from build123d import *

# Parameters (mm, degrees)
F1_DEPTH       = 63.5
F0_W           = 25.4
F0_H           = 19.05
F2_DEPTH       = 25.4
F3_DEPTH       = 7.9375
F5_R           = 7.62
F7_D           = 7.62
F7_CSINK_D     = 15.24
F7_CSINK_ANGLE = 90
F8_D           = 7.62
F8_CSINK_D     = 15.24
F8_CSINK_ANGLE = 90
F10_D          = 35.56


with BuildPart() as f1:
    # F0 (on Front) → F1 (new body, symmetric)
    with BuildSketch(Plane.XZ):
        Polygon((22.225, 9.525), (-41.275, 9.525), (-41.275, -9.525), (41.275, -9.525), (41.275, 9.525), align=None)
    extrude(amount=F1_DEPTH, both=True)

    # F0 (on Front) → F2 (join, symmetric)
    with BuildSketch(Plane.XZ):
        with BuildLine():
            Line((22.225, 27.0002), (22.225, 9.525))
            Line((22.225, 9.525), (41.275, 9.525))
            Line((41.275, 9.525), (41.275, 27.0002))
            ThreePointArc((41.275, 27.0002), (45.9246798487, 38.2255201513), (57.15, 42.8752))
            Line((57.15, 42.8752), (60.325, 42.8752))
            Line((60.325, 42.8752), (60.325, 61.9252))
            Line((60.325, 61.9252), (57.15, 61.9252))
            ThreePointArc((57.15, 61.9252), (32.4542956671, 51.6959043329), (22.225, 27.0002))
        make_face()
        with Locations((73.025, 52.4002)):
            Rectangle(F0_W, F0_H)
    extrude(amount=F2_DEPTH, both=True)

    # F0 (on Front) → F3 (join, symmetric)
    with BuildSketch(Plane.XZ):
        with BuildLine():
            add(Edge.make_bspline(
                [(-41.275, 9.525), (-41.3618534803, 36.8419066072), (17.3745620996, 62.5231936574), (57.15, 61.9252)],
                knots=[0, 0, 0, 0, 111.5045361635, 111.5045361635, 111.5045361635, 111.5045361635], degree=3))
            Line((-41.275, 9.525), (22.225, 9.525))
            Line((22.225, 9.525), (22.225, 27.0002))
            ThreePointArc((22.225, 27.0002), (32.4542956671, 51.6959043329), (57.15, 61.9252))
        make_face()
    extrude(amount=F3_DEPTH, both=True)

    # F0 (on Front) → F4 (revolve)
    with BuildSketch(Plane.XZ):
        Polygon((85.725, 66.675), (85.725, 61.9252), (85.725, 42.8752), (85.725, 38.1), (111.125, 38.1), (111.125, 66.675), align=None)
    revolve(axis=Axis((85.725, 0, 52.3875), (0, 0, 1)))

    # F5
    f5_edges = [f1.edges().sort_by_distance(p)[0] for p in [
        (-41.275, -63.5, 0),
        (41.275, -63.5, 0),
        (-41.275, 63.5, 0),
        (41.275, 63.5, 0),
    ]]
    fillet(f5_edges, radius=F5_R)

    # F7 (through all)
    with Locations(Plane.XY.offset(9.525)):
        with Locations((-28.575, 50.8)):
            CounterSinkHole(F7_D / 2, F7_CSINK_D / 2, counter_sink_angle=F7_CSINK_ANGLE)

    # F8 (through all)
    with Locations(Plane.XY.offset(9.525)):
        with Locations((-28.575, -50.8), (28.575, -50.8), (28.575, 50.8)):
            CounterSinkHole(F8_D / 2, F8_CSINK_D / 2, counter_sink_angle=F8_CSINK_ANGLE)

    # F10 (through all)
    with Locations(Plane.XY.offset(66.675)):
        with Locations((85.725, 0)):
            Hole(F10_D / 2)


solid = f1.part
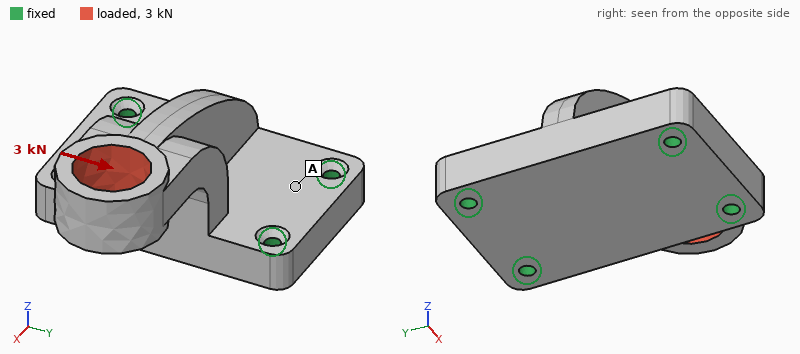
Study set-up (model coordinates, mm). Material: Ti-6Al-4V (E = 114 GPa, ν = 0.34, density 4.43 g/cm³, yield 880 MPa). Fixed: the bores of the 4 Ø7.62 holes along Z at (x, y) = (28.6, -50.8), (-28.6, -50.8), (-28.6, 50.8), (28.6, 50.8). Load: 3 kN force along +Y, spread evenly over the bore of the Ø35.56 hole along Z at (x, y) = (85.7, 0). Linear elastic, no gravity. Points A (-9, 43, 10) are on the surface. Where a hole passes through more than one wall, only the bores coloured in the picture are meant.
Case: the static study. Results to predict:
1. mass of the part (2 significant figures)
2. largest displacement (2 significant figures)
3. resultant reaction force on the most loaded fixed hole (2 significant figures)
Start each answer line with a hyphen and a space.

- 1.4 kg
- 0.11 mm
- 2.5 kN
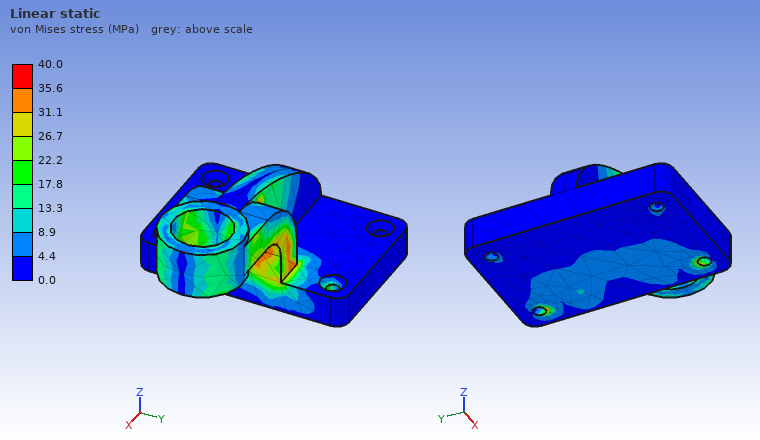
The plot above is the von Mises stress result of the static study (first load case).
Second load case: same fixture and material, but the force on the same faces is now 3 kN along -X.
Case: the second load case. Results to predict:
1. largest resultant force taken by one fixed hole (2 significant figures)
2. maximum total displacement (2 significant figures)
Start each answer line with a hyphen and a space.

- 1.7 kN
- 46 µm
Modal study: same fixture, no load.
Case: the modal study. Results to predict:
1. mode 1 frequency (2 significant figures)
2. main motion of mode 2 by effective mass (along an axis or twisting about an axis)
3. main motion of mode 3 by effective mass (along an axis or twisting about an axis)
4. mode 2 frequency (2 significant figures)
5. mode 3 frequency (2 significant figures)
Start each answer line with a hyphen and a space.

- 2000 Hz
- along Y
- along X
- 2300 Hz
- 4300 Hz
